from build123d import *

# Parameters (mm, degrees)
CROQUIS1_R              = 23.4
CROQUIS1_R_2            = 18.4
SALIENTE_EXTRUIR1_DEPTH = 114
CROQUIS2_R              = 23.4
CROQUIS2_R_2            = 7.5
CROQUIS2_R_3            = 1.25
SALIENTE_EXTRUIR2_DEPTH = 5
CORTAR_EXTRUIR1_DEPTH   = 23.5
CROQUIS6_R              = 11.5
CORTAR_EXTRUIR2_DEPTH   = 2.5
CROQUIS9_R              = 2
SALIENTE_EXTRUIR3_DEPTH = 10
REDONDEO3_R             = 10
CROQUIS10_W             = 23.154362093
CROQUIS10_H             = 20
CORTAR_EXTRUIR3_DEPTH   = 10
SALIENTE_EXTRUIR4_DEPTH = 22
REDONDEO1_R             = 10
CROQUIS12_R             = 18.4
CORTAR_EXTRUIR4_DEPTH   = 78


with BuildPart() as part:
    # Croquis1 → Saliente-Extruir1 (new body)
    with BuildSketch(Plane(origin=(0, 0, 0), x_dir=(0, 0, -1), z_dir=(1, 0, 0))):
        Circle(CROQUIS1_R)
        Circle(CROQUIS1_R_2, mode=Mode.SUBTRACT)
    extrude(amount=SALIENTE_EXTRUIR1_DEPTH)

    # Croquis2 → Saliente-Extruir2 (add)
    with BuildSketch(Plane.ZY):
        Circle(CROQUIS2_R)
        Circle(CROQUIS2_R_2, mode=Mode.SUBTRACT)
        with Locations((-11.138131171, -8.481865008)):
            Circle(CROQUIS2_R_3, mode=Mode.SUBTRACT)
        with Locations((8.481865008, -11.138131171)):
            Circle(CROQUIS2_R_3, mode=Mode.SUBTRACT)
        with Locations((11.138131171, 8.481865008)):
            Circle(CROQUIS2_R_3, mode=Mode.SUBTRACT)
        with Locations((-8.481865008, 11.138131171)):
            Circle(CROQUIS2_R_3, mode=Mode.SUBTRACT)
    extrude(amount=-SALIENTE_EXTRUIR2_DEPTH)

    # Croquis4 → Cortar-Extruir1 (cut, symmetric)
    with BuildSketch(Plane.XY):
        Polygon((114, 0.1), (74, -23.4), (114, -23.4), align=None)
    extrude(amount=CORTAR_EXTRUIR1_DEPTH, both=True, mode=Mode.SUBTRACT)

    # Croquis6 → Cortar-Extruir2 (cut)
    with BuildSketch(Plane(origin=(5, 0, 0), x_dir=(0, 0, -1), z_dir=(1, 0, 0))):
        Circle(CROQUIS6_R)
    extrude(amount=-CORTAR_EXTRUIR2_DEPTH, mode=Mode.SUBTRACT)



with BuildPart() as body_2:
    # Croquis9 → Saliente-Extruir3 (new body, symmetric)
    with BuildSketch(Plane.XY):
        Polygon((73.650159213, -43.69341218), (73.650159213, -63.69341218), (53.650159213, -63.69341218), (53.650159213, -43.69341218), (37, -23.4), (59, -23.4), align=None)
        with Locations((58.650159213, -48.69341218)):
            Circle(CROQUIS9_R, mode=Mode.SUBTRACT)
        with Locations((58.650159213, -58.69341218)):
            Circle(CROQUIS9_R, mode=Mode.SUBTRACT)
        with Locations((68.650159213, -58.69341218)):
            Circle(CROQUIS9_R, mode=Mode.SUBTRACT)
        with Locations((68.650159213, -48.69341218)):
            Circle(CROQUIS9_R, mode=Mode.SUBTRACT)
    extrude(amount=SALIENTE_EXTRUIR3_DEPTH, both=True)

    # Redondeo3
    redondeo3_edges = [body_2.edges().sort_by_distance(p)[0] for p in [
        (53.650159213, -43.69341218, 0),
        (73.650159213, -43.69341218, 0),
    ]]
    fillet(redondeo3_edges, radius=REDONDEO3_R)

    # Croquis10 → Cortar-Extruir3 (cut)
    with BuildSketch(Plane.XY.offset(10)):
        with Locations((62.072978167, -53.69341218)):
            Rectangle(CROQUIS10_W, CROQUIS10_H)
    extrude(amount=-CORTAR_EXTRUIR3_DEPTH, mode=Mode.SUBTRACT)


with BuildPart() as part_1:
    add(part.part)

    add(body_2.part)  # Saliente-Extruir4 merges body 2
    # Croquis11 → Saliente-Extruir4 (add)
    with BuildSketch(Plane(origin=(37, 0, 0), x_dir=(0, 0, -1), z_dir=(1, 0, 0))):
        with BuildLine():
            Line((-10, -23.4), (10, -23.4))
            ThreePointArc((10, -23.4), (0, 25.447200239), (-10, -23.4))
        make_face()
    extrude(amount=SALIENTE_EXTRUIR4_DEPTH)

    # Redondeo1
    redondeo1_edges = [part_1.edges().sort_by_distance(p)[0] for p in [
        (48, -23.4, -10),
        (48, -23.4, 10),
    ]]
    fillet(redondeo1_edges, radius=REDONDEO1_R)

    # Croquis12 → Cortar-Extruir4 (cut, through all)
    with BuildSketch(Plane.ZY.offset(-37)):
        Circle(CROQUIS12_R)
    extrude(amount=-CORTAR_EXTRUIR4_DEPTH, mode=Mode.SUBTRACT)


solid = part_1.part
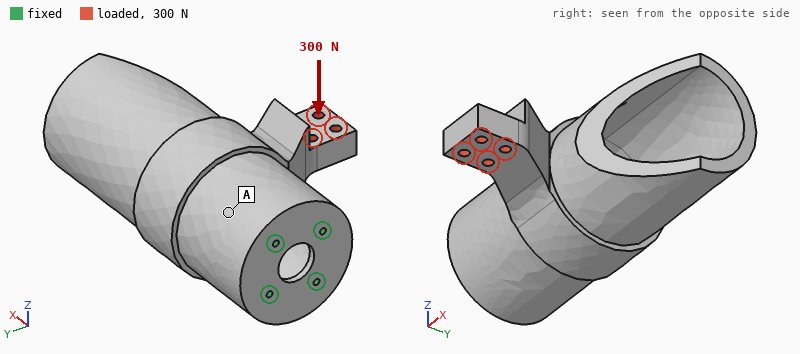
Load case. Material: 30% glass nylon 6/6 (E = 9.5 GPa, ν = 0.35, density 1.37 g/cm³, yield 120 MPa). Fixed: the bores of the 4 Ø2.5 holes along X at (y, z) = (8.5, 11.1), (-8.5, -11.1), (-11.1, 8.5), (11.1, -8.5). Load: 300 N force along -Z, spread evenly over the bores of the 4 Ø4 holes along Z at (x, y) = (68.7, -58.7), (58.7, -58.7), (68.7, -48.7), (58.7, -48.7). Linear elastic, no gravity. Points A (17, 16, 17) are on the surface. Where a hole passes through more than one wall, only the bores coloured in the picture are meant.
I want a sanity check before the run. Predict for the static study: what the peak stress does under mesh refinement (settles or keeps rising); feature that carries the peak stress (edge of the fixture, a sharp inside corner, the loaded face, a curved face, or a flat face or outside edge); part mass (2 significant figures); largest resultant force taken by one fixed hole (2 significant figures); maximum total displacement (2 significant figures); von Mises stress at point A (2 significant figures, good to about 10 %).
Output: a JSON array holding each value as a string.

["keeps rising", "edge of the fixture", "120 g", "550 N", "0.39 mm", "2.5 MPa"]
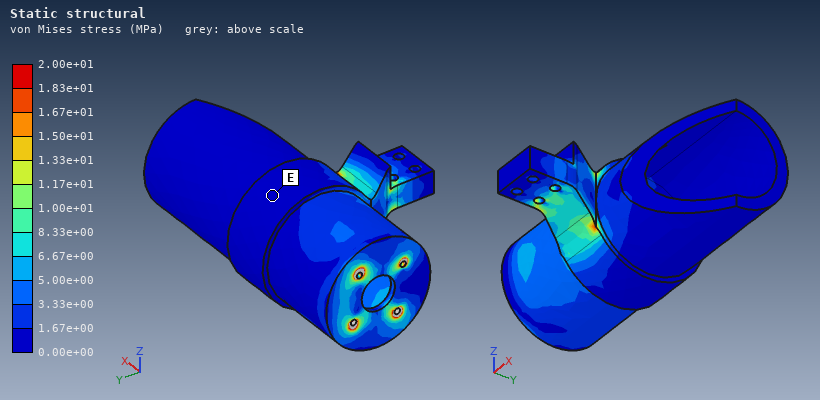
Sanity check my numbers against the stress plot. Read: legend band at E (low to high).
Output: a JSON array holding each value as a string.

["0.00e+00 to 1.67e+00 MPa"]
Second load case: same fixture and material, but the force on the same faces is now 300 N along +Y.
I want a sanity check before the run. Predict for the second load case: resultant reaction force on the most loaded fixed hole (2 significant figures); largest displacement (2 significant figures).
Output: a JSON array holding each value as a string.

["420 N", "0.29 mm"]
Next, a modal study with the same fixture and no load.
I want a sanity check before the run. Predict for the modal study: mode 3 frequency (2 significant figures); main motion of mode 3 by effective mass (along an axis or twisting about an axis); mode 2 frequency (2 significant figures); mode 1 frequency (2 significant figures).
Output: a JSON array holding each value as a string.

["2300 Hz", "twisting about X", "700 Hz", "680 Hz"]
